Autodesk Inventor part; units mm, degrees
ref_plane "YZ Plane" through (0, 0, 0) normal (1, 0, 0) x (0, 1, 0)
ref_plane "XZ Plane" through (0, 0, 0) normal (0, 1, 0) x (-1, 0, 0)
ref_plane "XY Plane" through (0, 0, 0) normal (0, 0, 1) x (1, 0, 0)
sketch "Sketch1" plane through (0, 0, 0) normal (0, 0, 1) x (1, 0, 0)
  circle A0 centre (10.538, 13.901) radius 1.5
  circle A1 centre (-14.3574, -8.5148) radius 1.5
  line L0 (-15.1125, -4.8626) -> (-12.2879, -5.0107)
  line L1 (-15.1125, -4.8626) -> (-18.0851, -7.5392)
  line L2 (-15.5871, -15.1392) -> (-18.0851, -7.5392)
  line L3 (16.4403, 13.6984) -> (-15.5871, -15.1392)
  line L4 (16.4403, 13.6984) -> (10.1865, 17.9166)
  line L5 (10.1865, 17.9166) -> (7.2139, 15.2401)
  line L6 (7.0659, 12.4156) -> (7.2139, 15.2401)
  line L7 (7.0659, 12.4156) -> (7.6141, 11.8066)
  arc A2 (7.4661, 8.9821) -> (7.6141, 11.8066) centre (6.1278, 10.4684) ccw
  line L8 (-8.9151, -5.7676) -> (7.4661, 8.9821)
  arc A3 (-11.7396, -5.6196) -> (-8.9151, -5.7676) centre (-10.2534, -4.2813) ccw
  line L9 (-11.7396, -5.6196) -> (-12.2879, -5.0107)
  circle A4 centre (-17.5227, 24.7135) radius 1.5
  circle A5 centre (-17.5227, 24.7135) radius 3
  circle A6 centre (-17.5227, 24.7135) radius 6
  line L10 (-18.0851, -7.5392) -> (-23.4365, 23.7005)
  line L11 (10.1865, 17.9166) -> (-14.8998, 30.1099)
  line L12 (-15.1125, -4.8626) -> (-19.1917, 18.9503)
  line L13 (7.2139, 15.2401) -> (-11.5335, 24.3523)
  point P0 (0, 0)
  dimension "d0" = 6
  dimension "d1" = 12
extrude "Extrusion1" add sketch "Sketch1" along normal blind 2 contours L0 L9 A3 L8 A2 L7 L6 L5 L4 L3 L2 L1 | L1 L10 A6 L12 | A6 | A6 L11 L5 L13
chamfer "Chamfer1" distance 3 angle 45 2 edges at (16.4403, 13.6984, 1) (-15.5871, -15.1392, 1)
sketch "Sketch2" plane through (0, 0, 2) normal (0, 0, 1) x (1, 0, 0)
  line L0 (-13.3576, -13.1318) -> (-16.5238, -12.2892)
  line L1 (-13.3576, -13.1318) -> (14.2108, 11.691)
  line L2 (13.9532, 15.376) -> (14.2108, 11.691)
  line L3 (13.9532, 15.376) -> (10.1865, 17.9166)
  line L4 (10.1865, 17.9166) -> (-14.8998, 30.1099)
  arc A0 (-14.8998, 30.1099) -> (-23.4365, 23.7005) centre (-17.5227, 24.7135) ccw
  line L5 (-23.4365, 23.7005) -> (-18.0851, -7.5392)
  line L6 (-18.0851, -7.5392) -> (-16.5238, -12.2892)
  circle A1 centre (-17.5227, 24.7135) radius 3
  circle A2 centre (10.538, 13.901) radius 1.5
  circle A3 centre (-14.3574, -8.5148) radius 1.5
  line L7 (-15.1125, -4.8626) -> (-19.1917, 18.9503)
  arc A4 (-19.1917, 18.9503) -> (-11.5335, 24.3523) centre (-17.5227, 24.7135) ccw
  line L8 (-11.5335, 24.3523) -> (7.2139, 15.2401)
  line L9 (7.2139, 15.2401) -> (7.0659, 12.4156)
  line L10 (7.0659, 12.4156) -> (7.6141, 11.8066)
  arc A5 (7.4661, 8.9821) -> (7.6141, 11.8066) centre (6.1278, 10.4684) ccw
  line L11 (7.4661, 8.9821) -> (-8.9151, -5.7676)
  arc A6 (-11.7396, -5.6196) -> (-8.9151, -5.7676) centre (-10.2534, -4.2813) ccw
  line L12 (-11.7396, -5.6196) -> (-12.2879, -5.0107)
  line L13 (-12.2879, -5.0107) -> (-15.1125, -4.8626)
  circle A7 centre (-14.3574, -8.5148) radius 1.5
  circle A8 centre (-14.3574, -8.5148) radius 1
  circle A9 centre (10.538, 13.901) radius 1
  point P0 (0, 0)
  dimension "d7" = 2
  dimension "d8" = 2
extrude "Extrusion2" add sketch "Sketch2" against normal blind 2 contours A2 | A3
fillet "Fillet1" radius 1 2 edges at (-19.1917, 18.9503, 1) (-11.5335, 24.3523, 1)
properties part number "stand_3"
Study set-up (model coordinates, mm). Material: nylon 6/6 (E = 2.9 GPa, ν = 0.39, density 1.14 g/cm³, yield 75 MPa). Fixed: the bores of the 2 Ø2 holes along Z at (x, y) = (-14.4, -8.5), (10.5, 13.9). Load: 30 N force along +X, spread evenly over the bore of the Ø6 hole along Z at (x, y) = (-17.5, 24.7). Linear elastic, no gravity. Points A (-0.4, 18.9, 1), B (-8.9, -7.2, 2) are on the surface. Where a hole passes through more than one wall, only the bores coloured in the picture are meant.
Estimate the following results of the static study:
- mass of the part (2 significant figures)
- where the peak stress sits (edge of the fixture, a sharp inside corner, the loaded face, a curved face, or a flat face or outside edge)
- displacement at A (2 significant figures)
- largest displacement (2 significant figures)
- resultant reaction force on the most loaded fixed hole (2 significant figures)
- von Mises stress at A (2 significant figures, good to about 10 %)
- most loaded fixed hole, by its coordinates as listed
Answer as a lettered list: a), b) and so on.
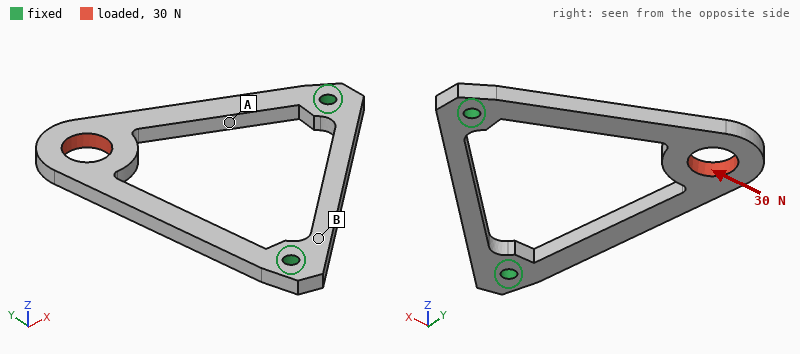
a) 0.95 g
b) a curved face
c) 0.11 mm
d) 0.23 mm
e) 30 N
f) 5.2 MPa
g) (10.5, 13.9)
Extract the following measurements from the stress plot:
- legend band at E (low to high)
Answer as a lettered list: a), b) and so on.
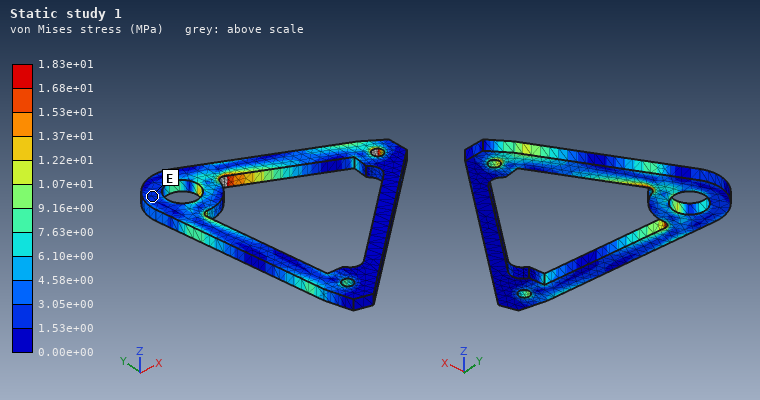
a) 1.53e+00 to 3.05e+00 MPa
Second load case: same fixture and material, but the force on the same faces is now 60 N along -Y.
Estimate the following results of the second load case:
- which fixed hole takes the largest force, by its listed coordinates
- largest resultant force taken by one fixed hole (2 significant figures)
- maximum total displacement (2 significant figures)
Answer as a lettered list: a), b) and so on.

a) (-14.4, -8.5)
b) 55 N
c) 0.36 mm
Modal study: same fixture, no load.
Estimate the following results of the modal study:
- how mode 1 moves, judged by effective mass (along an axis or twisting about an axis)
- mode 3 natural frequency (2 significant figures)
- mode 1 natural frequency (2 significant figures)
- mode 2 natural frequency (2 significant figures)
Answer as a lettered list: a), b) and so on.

a) along Z
b) 2500 Hz
c) 430 Hz
d) 1800 Hz
